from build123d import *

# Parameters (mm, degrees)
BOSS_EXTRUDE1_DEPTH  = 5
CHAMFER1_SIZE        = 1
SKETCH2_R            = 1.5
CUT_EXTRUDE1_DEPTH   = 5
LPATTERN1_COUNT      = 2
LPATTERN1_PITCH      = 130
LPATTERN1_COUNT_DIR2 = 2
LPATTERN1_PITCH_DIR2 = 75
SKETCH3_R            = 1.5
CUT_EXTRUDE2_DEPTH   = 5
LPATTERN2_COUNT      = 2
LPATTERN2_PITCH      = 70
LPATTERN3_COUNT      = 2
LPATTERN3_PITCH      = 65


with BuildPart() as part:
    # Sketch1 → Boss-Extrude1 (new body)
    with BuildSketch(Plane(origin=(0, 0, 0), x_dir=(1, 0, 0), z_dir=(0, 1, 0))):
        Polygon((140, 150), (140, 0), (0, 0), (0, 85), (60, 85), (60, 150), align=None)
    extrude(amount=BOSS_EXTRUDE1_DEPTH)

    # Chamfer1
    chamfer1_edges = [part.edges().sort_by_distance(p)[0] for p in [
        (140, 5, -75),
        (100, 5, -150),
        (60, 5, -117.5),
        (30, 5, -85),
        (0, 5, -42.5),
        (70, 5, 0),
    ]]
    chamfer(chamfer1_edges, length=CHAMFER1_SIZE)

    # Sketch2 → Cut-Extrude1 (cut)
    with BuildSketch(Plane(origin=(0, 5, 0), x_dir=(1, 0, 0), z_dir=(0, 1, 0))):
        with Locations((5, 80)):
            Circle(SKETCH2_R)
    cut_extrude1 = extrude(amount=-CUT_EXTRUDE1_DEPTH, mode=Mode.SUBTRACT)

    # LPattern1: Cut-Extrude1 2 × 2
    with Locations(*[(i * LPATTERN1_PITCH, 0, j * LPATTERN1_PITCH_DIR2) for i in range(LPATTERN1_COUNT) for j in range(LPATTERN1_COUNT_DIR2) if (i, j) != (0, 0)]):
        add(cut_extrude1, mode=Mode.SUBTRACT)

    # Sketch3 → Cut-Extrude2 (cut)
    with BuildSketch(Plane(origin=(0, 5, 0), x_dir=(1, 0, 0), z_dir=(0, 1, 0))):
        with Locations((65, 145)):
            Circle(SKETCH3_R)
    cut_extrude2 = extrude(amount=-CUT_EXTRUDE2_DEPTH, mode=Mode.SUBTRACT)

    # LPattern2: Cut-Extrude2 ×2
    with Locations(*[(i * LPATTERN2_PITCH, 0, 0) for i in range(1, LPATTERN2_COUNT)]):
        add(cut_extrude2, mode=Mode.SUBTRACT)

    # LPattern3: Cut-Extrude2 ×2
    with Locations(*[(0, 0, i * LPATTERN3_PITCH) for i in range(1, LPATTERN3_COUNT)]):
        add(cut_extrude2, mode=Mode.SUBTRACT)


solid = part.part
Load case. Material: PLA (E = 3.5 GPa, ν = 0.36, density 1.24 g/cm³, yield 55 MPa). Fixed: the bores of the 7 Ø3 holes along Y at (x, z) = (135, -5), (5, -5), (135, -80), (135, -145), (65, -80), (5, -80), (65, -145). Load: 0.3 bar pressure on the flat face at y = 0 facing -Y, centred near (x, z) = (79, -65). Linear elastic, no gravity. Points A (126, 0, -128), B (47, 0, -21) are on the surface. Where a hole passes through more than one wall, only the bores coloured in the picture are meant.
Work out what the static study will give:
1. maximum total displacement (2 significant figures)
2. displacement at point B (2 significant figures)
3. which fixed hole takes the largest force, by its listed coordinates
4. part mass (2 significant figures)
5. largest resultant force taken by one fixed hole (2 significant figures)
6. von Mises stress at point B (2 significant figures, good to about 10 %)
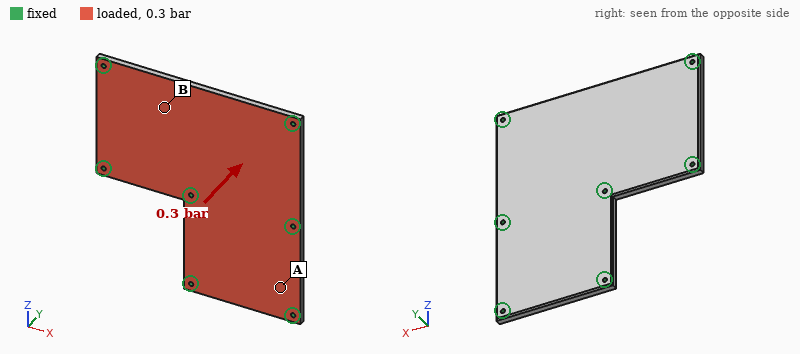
0.76 mm
0.49 mm
(65, -80)
110 g
160 N
3.6 MPa
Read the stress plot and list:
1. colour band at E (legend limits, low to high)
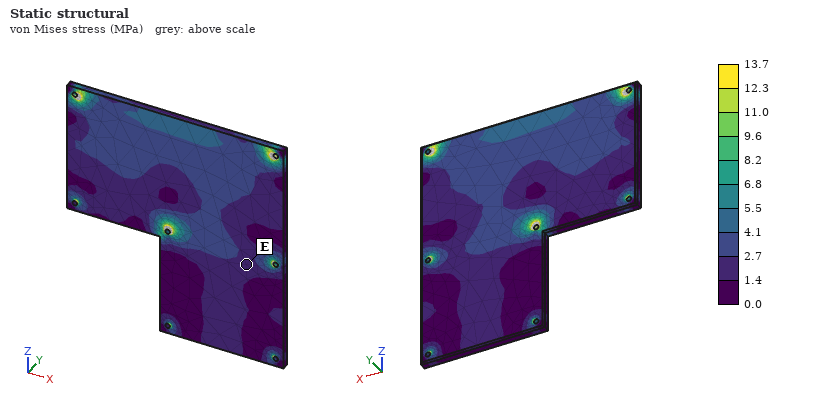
1.4 to 2.7 MPa
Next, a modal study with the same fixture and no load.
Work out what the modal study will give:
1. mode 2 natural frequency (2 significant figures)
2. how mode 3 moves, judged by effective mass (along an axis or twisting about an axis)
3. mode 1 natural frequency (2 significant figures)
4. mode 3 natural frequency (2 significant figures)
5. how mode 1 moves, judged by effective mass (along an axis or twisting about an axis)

1100 Hz
along Y
530 Hz
1200 Hz
along Y
